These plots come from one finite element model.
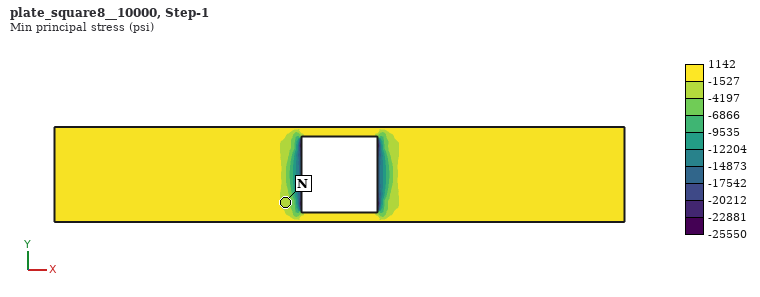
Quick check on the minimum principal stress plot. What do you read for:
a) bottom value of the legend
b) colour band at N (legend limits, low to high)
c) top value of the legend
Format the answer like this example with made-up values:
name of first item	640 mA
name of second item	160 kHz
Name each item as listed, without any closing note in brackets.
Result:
bottom value of the legend	-25550 psi
colour band at N	-4197 to -1527 psi
top value of the legend	1142 psi
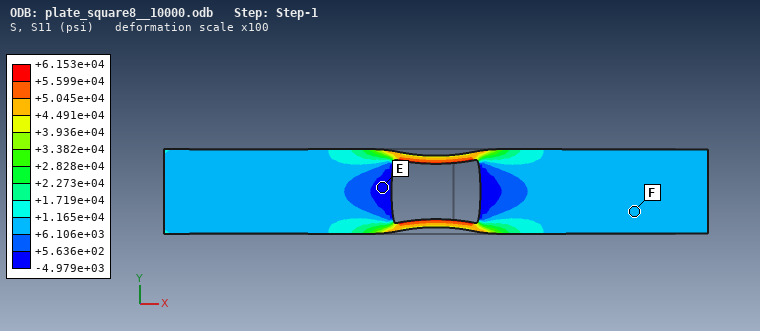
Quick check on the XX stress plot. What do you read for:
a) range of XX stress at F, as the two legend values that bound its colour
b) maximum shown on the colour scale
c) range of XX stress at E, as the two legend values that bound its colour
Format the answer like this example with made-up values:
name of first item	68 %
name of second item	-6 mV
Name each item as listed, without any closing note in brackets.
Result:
range of XX stress at F, as the two legend values that bound its colour	+6.106e+03 to +1.165e+04 psi
maximum shown on the colour scale	+6.153e+04 psi
range of XX stress at E, as the two legend values that bound its colour	-4.979e+03 to +5.636e+02 psi
